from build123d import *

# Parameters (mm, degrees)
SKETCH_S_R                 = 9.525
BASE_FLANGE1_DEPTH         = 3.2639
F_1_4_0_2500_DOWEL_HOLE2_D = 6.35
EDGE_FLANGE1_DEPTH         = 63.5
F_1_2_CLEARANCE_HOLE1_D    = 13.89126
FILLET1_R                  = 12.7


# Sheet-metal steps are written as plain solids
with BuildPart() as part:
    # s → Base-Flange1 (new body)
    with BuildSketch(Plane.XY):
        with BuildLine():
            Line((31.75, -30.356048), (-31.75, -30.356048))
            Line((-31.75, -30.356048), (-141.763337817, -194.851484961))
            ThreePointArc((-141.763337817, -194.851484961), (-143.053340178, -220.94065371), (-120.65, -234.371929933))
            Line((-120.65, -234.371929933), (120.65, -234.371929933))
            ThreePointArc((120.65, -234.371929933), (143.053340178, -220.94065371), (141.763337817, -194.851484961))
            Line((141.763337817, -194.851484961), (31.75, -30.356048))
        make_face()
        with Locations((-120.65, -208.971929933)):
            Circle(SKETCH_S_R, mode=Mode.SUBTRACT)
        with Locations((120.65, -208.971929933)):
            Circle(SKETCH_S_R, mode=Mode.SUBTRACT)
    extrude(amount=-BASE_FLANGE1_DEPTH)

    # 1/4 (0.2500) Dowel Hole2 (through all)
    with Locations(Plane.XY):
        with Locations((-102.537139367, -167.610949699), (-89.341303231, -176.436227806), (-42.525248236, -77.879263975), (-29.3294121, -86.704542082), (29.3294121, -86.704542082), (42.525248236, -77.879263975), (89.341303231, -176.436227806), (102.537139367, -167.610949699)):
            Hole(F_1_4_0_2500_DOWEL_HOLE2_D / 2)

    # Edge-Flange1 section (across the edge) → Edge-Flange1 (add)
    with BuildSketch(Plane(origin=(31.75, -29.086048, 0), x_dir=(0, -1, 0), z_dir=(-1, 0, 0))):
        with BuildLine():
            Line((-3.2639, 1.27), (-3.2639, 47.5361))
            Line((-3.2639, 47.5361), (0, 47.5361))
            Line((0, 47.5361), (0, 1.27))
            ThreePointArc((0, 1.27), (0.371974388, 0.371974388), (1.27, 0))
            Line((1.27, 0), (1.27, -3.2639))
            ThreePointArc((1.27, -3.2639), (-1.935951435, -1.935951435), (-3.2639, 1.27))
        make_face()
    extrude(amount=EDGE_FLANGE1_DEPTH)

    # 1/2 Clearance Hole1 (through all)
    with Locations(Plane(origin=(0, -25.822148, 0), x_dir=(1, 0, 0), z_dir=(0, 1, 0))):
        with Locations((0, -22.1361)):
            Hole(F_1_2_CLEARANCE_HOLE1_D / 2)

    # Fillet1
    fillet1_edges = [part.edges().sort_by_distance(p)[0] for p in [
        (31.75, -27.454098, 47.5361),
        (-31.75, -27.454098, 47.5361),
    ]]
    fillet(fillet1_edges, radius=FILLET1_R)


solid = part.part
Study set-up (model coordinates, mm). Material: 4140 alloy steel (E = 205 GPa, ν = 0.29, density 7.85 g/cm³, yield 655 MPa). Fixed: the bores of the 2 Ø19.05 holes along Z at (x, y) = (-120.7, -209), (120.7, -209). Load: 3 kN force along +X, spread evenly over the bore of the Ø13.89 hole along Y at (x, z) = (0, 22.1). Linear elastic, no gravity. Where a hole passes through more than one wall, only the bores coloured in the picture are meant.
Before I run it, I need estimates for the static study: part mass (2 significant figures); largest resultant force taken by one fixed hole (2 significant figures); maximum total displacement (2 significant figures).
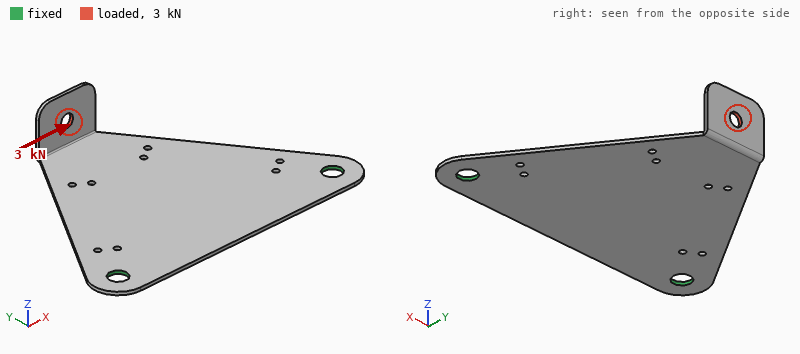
1.1 kg
2.7 kN
4.3 mm
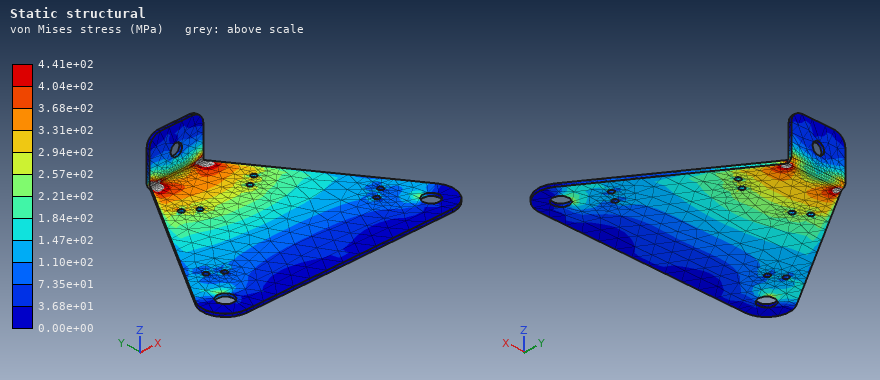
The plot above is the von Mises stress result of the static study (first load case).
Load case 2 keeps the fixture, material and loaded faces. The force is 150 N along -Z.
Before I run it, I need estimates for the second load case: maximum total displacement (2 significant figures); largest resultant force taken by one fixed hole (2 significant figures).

3.7 mm
75 N
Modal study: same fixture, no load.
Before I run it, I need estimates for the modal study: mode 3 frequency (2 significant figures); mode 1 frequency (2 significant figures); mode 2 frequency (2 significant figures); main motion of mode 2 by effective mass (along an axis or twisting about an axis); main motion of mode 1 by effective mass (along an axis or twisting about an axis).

310 Hz
74 Hz
290 Hz
along Z
along Z
